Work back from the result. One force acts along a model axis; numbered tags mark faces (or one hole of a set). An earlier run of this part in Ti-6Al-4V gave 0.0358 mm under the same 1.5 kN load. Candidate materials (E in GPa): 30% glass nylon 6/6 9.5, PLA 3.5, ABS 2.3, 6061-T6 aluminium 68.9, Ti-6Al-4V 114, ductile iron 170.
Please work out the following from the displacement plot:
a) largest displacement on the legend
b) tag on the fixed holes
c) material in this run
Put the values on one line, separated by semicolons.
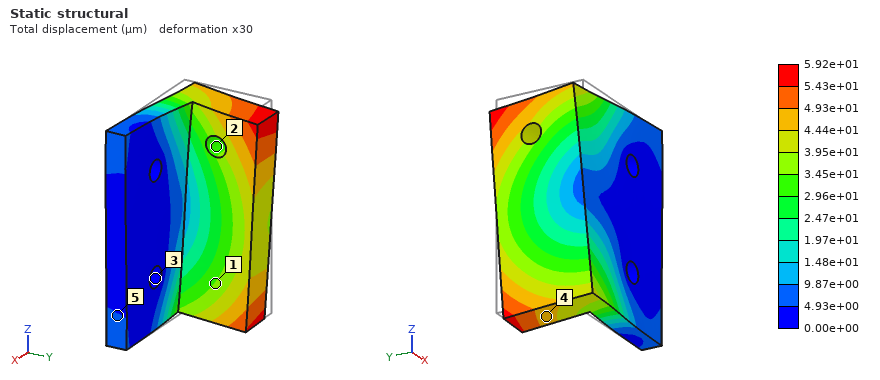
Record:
5.92e+01 µm; 3; 6061-T6 aluminium
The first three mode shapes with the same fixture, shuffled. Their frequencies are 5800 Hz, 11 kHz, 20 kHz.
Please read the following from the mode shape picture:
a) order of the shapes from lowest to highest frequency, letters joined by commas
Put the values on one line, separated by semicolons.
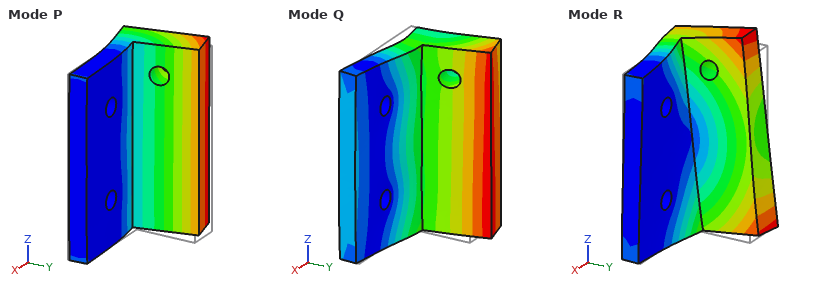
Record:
P, R, Q
